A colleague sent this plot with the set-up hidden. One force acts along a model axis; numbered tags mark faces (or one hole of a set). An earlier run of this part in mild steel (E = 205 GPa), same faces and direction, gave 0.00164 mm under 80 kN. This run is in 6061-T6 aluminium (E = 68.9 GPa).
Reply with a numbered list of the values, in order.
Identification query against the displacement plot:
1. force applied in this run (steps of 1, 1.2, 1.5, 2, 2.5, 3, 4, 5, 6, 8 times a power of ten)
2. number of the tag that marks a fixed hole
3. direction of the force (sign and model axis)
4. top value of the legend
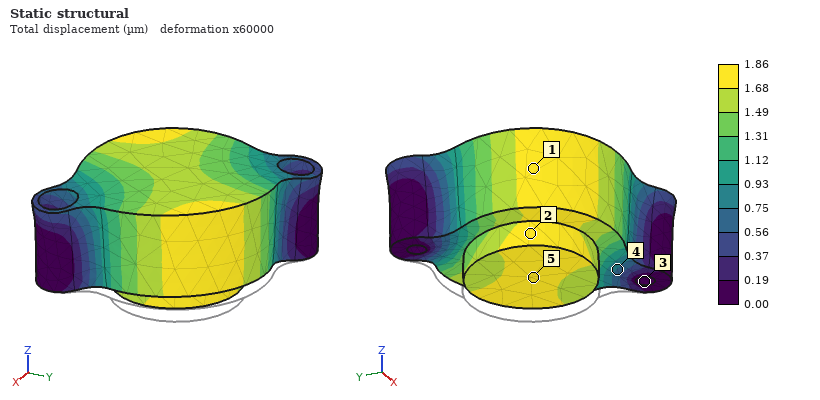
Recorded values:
1. 30 kN
2. 3
3. +Z
4. 1.86 µm
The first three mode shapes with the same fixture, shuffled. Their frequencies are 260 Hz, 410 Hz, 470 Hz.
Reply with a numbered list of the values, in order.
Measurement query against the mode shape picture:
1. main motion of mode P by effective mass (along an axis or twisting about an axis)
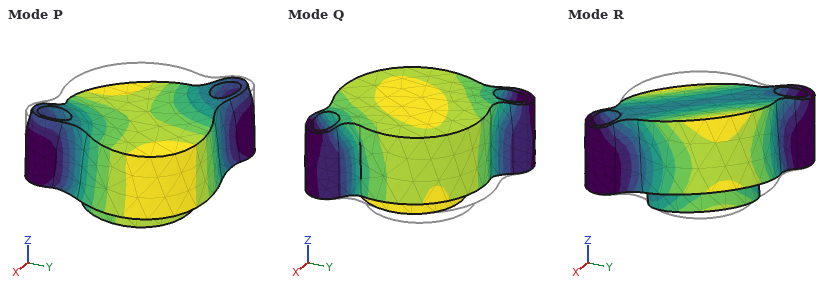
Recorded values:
1. along Z
